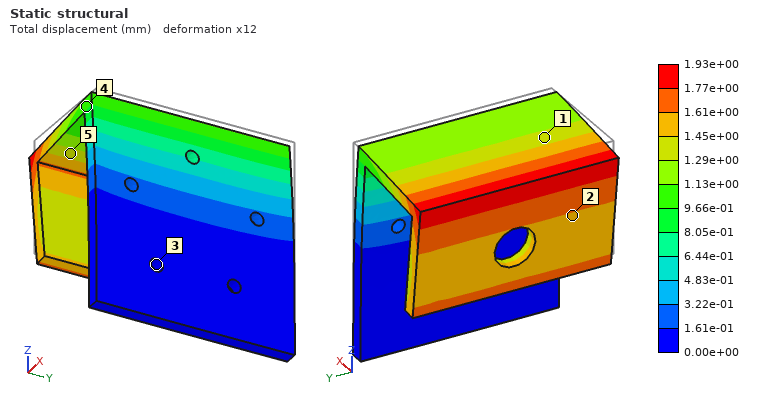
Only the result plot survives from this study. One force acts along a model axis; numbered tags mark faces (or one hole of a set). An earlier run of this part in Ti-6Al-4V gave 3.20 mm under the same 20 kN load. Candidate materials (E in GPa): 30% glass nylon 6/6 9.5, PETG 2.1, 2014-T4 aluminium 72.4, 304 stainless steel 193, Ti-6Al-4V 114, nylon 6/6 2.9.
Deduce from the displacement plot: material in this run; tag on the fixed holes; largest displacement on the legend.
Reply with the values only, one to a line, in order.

304 stainless steel
3
1.93e+00 mm
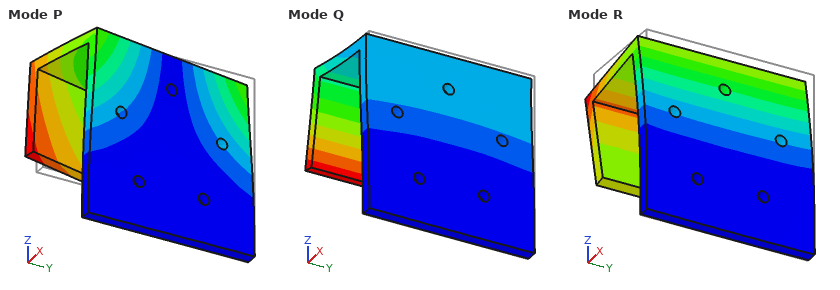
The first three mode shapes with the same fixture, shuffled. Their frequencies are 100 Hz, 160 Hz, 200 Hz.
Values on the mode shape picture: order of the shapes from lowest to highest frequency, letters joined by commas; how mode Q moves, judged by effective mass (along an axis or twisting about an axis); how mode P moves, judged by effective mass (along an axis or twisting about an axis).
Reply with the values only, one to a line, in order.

R, P, Q
along X
along Y
